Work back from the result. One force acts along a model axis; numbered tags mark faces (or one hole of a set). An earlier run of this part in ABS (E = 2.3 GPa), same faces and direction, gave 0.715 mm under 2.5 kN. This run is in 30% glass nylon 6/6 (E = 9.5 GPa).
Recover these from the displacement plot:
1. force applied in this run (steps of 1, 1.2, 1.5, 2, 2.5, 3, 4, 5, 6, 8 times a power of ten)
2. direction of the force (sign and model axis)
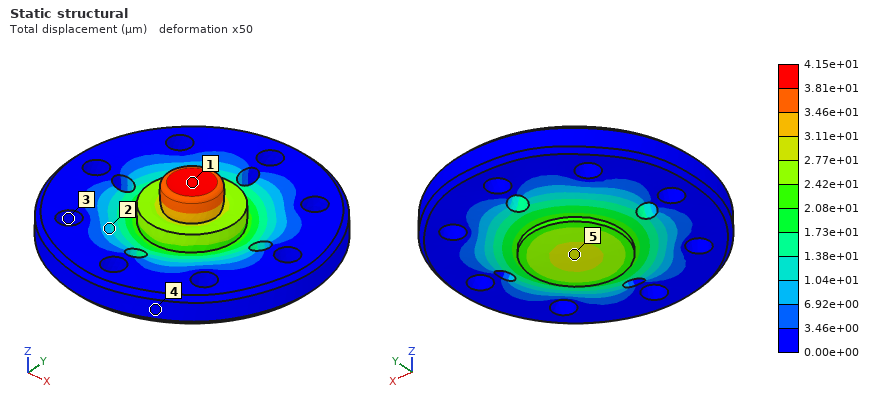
600 N
-Z
